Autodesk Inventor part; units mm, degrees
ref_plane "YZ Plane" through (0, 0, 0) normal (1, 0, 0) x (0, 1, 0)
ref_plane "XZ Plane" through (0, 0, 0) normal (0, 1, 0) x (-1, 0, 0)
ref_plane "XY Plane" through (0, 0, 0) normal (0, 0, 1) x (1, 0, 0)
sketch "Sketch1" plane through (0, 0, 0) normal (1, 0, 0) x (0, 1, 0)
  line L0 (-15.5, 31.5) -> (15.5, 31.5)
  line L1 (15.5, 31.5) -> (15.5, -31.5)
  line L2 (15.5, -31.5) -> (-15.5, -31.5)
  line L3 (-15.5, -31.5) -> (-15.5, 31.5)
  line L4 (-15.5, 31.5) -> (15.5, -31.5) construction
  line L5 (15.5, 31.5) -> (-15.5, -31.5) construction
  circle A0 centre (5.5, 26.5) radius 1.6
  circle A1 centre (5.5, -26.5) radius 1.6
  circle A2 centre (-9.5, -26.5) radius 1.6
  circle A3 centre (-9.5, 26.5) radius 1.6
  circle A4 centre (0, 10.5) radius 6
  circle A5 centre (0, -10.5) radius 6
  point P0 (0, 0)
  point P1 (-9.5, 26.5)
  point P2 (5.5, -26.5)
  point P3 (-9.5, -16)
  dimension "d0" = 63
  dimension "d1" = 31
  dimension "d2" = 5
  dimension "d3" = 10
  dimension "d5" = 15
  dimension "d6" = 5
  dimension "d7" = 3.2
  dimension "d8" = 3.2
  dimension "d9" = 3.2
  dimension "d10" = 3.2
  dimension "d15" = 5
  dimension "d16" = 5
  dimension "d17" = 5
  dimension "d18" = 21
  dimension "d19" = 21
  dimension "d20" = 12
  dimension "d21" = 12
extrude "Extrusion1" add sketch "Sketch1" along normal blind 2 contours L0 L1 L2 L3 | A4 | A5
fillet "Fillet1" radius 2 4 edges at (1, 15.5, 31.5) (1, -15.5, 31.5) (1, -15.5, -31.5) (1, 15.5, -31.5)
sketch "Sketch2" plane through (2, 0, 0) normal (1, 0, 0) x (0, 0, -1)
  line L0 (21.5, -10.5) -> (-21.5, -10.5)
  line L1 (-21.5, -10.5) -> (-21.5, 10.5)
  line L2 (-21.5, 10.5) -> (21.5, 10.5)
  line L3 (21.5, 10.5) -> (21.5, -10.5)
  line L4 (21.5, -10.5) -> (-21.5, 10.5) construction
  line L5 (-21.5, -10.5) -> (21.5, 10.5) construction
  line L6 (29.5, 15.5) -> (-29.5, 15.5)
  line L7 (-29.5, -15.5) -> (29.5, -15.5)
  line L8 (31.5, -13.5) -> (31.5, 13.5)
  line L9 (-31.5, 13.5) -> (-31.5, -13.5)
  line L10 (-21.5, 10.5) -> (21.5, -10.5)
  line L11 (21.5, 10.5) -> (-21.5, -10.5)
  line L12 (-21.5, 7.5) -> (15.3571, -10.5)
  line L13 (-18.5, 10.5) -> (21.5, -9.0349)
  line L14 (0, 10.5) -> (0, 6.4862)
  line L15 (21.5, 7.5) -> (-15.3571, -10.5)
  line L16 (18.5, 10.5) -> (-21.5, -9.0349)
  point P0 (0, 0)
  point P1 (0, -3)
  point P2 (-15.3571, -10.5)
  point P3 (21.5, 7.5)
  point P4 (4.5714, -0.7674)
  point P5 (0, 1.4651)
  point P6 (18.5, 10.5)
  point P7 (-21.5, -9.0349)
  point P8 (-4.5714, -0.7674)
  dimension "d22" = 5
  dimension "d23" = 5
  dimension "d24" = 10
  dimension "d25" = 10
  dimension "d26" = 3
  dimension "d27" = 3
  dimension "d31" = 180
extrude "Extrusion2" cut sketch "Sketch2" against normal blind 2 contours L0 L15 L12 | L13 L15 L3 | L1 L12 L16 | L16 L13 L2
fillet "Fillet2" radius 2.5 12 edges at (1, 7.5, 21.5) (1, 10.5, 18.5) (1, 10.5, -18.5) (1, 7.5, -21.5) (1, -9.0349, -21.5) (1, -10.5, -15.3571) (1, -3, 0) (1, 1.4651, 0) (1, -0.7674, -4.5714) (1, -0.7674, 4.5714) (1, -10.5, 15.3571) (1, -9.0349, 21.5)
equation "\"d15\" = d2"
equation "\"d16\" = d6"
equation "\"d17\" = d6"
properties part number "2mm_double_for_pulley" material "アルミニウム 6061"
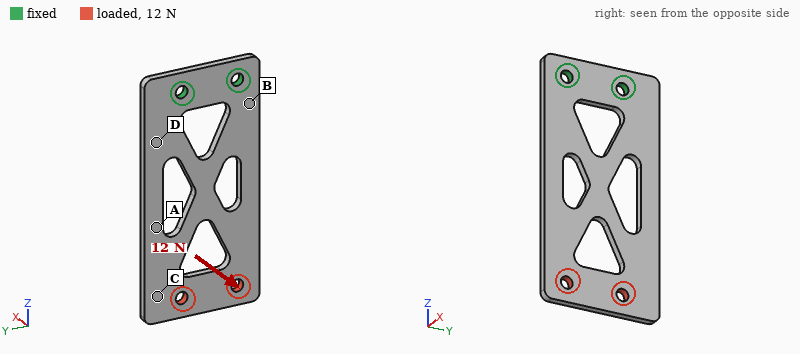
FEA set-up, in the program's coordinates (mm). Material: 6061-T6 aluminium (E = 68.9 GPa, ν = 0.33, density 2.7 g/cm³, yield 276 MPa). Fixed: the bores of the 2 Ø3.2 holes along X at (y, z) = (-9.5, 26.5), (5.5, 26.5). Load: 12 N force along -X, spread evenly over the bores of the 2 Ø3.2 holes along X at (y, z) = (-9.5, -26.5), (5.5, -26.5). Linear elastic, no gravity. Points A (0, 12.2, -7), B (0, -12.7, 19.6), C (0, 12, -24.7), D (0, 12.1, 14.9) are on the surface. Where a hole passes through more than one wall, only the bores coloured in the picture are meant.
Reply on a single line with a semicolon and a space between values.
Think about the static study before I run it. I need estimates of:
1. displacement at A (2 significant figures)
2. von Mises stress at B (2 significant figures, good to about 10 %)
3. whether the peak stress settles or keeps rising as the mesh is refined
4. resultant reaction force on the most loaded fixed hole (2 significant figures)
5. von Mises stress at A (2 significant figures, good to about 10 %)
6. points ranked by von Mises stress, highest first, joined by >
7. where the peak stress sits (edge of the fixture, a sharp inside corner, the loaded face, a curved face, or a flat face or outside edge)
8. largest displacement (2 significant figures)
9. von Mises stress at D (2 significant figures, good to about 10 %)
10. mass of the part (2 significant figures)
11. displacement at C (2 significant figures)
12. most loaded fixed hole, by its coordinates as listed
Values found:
0.30 mm; 46 MPa; keeps rising; 7.1 N; 22 MPa; B > D > A > C; edge of the fixture; 0.76 mm; 34 MPa; 7.9 g; 0.62 mm; (-9.5, 26.5)
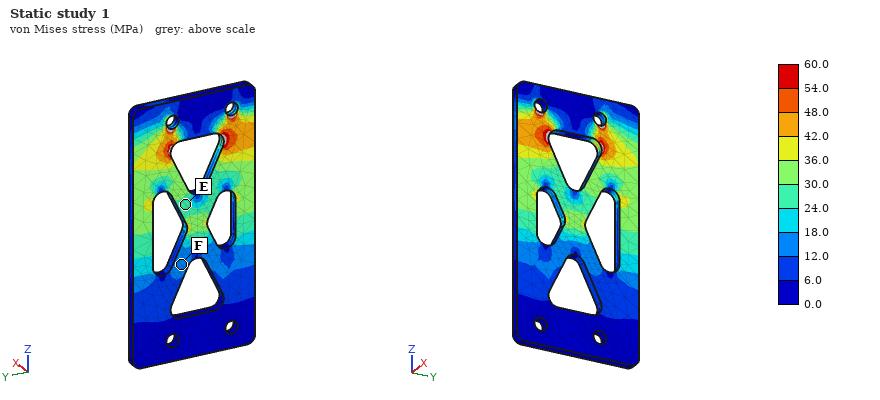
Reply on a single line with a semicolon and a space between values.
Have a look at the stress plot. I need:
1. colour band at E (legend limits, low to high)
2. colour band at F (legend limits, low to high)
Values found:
24.0 to 30.0 MPa; 12.0 to 18.0 MPa
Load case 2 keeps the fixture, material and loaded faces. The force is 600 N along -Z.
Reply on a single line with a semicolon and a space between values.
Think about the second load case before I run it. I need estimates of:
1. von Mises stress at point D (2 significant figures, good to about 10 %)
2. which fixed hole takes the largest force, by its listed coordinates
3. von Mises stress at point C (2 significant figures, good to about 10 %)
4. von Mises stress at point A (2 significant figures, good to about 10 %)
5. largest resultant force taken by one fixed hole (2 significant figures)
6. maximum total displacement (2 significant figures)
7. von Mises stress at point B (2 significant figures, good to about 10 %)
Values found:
13 MPa; (-9.5, 26.5); 8.0 MPa; 18 MPa; 320 N; 20 µm; 16 MPa
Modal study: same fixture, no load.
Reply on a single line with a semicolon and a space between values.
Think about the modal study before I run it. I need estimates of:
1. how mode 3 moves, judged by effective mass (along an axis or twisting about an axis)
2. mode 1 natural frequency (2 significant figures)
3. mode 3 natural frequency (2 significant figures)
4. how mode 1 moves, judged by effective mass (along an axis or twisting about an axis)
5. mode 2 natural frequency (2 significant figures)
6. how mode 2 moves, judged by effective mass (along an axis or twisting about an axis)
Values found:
along X; 430 Hz; 2800 Hz; along X; 1600 Hz; twisting about Z
